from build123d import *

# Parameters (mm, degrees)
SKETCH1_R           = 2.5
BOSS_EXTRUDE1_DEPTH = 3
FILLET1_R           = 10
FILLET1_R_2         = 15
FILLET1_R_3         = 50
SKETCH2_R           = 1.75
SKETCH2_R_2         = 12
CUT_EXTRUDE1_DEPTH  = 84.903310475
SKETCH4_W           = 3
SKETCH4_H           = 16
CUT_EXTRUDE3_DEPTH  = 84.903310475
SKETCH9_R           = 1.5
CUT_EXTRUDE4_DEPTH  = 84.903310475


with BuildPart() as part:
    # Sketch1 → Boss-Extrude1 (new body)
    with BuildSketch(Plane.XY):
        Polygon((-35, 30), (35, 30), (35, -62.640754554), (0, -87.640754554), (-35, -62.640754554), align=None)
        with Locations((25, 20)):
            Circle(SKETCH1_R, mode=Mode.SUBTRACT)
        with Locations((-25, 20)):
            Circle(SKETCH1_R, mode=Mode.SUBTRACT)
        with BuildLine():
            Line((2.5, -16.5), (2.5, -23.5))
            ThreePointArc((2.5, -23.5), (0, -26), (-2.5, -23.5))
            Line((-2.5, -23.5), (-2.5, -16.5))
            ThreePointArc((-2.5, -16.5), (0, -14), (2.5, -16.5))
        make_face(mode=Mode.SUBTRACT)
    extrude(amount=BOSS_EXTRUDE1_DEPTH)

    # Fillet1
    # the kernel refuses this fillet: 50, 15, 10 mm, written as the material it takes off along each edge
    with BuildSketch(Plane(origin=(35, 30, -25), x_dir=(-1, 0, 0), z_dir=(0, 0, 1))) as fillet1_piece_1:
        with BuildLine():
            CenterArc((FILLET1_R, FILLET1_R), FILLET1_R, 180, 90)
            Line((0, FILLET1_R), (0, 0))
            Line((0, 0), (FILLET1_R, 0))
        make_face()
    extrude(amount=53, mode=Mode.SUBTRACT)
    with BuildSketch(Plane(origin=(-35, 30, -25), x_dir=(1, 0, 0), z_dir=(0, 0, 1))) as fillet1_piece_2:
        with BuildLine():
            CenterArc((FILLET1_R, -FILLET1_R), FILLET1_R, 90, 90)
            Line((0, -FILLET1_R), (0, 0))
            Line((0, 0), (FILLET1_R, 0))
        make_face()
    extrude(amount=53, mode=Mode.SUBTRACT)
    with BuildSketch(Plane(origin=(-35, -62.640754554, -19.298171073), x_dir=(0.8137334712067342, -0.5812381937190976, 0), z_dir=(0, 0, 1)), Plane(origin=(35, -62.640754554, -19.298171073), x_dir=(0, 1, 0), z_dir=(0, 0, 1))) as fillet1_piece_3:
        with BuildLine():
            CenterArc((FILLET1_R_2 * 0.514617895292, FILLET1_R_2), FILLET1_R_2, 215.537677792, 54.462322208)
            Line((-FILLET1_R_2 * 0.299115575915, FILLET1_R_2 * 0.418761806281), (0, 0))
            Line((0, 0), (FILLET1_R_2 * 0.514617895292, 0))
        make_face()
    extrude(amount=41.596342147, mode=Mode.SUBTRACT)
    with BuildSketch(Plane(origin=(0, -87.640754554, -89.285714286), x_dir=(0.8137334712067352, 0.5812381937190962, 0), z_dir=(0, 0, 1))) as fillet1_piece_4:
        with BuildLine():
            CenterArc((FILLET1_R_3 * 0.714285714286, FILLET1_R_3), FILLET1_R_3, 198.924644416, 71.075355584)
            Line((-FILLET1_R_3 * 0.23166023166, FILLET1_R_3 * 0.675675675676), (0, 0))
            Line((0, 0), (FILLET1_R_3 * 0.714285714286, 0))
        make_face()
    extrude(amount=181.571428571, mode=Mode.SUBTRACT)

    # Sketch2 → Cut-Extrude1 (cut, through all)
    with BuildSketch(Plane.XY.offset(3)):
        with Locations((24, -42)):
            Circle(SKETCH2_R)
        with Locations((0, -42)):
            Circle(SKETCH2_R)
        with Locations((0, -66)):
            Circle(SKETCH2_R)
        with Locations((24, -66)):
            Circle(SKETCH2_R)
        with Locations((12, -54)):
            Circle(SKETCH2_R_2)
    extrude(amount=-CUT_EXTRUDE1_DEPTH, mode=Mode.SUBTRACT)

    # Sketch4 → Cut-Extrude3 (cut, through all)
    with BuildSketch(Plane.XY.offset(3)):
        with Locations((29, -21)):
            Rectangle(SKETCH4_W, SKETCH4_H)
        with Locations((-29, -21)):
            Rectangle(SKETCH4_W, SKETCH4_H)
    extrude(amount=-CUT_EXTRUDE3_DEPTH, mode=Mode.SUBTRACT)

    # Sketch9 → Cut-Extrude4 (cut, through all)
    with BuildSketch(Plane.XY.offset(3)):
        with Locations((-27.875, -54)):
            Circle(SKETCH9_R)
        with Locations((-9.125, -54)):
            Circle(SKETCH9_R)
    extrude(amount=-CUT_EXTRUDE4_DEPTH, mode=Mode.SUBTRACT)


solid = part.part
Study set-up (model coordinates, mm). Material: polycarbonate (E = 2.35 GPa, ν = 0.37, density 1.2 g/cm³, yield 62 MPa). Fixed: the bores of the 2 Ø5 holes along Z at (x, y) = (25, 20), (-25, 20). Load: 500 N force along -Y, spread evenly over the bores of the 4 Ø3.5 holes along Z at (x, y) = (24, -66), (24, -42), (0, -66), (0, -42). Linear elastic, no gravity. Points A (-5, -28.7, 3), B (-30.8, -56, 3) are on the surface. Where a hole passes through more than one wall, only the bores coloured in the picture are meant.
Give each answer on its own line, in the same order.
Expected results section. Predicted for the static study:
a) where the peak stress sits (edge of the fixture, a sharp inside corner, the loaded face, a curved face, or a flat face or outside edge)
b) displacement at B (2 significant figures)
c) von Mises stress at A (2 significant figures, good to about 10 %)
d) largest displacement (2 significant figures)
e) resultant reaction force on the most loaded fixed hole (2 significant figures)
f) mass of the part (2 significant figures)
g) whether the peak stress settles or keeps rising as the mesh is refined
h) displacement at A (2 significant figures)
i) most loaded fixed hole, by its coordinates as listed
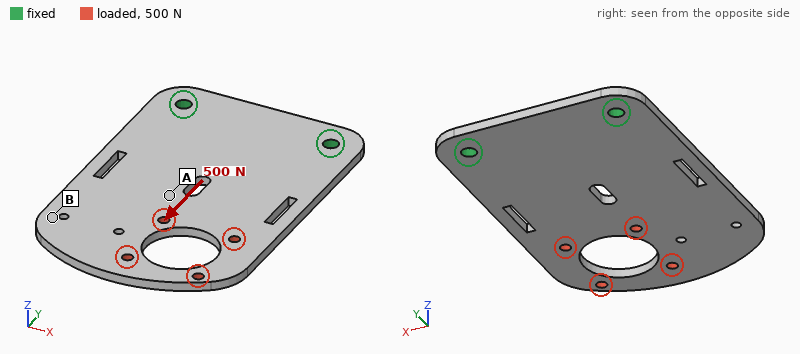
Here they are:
edge of the fixture
0.100 mm
3.3 MPa
0.27 mm
370 N
23 g
keeps rising
0.077 mm
(25, 20)
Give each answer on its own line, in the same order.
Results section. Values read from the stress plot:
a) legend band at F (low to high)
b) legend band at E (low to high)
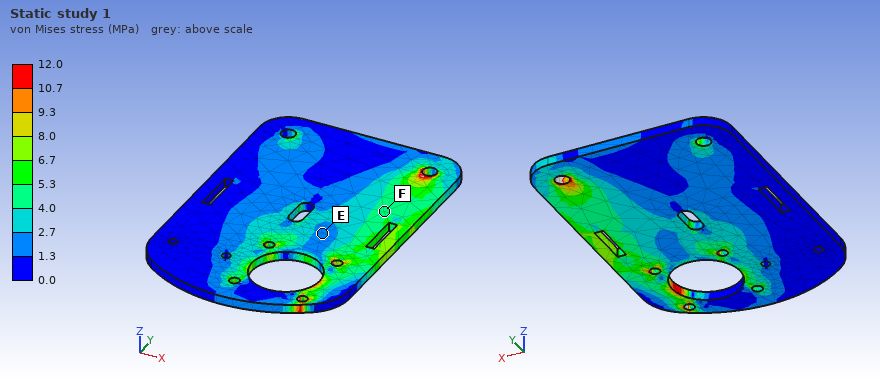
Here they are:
4.0 to 5.3 MPa
1.3 to 2.7 MPa
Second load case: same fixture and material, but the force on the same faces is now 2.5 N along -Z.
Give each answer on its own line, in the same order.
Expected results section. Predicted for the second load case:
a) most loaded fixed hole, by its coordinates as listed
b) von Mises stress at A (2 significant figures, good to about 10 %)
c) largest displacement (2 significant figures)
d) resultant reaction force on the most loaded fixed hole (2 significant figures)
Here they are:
(25, 20)
0.70 MPa
1.5 mm
1.8 N
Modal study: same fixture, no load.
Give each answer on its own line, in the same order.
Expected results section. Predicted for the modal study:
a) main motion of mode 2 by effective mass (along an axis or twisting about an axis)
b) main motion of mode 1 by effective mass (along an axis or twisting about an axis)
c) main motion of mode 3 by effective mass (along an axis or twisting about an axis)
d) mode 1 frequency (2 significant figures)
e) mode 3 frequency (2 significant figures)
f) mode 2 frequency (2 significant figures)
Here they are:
twisting about Y
along Z
along Z
85 Hz
470 Hz
260 Hz
